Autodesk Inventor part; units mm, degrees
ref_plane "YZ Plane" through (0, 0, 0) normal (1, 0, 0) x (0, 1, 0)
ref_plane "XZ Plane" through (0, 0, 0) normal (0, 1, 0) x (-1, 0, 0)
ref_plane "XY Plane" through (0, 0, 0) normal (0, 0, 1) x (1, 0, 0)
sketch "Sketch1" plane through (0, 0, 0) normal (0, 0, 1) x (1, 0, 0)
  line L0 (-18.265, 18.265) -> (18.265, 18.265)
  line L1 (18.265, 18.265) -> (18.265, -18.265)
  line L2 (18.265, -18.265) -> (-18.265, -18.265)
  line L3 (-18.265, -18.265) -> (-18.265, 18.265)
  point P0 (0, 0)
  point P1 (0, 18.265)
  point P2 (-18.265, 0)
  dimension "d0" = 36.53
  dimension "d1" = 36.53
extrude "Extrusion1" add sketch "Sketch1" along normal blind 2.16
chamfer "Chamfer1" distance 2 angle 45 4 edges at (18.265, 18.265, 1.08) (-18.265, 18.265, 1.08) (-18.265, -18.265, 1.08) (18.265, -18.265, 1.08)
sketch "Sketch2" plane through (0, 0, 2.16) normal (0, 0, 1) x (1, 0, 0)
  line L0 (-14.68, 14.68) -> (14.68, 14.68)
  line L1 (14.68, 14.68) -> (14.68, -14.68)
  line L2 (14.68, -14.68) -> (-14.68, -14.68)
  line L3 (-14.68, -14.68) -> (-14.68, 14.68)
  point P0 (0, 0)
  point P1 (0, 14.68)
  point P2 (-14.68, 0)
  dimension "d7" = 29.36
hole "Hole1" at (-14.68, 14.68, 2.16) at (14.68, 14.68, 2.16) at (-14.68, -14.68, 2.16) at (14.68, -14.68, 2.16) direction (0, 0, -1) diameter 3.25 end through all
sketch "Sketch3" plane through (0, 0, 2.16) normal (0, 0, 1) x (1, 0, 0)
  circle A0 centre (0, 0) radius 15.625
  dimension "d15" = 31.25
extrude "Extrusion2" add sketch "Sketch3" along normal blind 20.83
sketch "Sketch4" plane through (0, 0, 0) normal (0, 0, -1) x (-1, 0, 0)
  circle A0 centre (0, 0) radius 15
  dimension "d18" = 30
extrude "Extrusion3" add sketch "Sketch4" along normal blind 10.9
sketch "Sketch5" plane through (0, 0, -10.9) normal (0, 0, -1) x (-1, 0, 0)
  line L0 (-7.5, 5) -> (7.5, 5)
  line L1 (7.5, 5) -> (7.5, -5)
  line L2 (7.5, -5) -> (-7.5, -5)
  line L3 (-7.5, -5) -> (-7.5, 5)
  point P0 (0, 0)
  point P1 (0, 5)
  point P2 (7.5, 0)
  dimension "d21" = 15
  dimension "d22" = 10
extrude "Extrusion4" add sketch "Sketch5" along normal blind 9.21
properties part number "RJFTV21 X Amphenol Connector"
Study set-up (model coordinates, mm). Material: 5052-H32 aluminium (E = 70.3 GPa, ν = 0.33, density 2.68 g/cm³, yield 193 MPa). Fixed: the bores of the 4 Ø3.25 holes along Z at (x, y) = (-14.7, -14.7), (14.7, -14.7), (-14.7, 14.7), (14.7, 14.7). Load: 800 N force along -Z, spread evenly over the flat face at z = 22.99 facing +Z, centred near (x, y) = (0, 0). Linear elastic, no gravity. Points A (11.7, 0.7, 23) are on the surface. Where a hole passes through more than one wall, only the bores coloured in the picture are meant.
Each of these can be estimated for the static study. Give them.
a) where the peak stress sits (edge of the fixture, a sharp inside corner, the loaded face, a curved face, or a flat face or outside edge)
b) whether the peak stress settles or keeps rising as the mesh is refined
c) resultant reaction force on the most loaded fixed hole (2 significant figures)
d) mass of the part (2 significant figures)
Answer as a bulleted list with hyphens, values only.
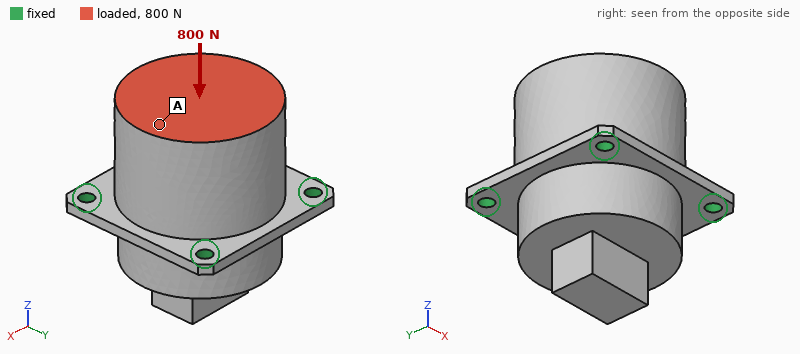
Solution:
- edge of the fixture
- keeps rising
- 200 N
- 75 g
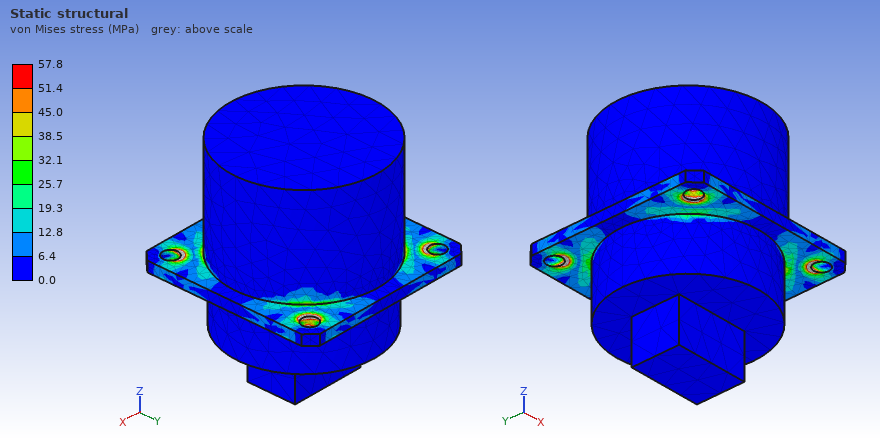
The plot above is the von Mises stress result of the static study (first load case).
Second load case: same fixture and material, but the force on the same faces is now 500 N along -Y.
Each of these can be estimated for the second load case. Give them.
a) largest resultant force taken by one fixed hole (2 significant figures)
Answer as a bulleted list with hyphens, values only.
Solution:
- 250 N
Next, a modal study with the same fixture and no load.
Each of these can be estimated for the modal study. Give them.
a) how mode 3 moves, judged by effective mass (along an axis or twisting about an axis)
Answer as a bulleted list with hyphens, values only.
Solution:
- along Z
